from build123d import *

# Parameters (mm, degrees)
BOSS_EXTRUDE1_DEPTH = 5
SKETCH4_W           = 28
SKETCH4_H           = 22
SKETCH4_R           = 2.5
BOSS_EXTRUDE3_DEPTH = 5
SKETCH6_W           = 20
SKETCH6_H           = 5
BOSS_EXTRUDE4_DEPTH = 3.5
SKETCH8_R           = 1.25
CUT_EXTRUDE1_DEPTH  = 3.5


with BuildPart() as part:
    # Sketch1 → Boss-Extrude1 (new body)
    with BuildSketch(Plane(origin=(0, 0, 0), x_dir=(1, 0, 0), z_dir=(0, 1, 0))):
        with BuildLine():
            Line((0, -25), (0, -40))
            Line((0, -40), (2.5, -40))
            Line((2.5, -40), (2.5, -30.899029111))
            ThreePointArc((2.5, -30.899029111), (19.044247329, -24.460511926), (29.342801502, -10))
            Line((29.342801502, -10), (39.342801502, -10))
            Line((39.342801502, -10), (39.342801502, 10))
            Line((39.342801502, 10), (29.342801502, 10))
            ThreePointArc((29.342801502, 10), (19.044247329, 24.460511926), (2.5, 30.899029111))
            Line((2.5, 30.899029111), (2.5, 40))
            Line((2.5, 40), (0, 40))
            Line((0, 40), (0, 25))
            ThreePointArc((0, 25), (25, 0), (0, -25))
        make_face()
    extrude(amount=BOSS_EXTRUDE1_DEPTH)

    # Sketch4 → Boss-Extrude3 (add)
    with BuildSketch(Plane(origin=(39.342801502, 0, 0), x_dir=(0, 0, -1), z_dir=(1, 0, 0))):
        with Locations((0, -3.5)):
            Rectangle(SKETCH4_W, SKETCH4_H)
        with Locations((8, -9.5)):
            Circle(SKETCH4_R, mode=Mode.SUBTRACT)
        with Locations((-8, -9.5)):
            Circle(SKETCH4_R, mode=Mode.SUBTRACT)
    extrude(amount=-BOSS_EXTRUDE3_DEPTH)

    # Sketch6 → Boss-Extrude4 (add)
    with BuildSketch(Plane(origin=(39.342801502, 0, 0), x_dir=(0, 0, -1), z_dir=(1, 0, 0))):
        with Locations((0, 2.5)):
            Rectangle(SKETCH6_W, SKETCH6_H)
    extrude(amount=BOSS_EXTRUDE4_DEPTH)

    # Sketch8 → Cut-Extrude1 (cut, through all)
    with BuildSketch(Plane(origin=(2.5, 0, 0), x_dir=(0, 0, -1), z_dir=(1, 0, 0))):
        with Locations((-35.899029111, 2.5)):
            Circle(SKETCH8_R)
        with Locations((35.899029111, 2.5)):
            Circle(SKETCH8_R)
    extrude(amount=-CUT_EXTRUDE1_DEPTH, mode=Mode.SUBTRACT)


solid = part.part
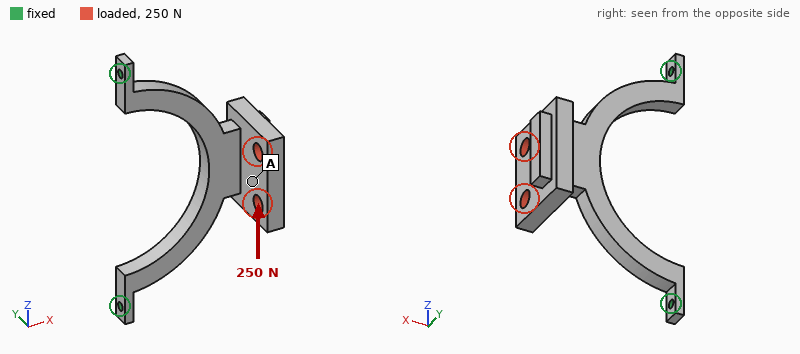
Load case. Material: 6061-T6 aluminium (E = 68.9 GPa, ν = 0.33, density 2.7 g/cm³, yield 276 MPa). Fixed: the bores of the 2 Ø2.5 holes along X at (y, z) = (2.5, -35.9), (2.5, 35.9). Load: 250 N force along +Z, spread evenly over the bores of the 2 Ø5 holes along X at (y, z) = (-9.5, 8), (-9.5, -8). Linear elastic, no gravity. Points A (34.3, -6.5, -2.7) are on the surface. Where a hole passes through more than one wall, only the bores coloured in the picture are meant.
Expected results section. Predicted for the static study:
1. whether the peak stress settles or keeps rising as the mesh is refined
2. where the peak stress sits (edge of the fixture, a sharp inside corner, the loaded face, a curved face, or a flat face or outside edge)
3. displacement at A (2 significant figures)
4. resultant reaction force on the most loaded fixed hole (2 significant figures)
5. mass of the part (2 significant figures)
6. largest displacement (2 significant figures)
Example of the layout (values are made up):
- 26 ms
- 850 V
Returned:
- keeps rising
- edge of the fixture
- 0.080 mm
- 190 N
- 17 g
- 0.16 mm
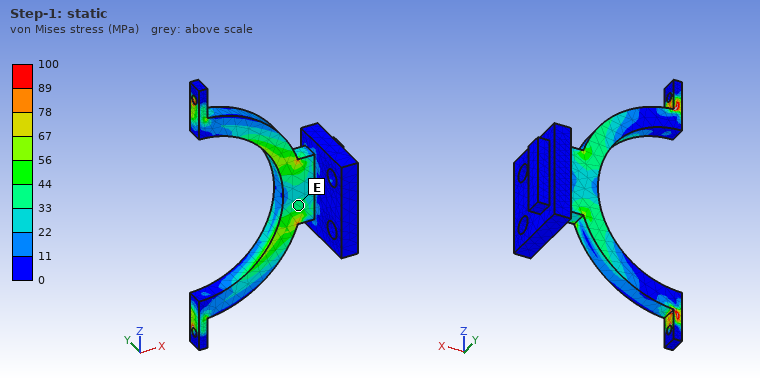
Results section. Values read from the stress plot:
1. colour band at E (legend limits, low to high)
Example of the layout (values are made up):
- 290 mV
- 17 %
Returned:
- 33 to 44 MPa
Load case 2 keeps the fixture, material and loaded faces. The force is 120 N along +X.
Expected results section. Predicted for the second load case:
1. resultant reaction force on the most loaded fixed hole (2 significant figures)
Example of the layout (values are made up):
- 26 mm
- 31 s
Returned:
- 77 N
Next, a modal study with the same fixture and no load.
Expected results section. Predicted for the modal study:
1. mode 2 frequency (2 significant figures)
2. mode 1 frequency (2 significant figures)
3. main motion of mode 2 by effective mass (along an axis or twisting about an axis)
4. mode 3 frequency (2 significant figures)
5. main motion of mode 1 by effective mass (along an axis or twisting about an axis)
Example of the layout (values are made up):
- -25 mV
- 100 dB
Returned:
- 2700 Hz
- 490 Hz
- along Z
- 3600 Hz
- along Y
